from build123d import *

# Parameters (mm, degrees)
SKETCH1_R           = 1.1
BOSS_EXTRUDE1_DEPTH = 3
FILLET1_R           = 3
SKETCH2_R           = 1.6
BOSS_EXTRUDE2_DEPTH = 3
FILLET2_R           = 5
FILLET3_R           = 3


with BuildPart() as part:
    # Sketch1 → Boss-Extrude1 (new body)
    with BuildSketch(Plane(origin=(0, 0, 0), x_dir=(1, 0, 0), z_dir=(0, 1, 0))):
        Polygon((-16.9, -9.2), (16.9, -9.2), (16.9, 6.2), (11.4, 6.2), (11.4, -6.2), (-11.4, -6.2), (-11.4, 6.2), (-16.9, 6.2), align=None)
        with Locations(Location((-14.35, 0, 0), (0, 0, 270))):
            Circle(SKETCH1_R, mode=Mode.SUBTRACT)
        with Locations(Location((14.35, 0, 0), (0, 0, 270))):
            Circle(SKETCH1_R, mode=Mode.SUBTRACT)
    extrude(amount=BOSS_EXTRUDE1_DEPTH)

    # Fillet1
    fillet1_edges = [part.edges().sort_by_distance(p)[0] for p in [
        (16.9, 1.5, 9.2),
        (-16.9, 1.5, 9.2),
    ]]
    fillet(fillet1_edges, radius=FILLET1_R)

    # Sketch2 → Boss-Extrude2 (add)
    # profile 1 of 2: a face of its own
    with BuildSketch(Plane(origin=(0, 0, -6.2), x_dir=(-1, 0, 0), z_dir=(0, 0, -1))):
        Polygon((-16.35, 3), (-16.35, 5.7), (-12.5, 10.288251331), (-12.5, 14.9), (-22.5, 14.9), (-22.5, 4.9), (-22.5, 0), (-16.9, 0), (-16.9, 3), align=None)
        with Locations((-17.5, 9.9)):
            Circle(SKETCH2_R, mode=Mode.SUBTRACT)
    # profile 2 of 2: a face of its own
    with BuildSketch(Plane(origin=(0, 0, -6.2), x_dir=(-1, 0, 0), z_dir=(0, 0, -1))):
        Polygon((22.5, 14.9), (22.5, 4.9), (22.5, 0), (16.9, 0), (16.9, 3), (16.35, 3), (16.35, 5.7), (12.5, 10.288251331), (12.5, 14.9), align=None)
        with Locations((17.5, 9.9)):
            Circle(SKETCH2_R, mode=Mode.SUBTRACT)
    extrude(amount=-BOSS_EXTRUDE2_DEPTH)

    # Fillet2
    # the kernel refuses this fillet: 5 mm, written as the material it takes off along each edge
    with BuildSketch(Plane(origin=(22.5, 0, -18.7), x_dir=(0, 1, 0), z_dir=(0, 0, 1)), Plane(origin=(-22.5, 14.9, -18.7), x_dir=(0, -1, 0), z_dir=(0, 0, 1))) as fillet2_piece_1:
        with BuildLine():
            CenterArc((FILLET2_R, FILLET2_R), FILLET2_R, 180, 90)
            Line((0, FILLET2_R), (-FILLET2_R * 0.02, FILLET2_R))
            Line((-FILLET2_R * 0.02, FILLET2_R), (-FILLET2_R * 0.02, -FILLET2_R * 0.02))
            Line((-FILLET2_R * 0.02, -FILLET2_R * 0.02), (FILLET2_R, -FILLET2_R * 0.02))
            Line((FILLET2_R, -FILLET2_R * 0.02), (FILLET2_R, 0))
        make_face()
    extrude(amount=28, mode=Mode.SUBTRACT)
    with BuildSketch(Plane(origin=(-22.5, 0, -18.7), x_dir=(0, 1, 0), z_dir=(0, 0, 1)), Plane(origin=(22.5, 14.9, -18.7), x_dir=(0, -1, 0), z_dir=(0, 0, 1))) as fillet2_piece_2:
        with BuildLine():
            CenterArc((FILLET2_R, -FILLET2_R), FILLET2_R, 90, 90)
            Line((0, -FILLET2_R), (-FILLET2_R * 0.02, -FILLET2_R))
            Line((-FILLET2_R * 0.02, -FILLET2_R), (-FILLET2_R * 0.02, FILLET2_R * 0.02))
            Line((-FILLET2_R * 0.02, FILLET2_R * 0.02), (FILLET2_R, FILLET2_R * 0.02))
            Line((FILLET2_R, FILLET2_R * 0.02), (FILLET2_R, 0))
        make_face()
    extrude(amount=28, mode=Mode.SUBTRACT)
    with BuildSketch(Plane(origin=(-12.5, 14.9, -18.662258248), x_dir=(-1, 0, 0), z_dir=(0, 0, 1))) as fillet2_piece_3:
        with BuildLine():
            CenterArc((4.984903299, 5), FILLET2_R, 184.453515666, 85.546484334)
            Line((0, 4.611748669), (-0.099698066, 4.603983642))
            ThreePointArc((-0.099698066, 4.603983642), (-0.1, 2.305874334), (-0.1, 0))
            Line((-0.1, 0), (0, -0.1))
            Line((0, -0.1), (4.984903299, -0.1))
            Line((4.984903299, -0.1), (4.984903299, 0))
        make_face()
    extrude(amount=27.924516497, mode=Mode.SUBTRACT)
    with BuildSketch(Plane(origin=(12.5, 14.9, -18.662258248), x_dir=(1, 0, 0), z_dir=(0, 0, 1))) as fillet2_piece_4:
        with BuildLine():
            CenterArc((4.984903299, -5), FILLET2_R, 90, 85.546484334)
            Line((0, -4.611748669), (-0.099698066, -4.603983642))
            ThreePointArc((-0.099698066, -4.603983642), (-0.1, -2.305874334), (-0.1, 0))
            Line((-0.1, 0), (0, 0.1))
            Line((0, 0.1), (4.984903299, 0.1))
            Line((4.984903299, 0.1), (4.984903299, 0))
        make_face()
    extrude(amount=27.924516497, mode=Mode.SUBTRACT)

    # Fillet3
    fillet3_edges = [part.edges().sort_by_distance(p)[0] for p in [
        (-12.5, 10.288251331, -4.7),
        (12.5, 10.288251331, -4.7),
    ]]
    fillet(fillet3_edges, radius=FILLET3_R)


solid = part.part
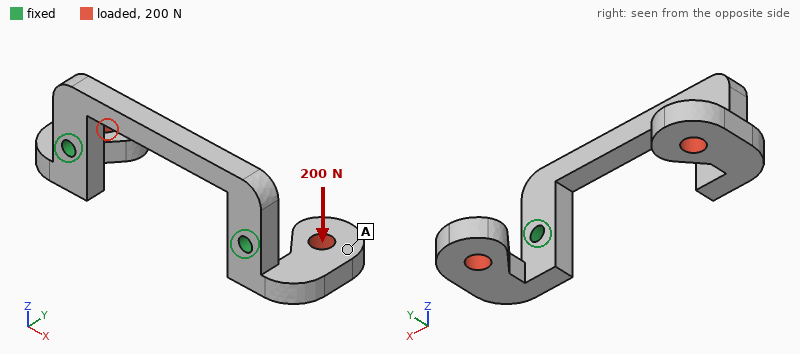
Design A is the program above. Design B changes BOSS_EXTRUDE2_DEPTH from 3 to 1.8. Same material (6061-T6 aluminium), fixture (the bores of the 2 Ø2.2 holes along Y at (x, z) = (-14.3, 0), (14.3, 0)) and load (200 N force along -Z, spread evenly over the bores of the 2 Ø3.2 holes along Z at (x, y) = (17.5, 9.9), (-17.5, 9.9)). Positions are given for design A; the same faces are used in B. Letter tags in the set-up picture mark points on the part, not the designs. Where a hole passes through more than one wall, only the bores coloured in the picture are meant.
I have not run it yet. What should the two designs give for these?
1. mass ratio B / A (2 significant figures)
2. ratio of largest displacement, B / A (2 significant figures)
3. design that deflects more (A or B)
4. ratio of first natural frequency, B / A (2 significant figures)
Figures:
0.82
2.5
B
0.84
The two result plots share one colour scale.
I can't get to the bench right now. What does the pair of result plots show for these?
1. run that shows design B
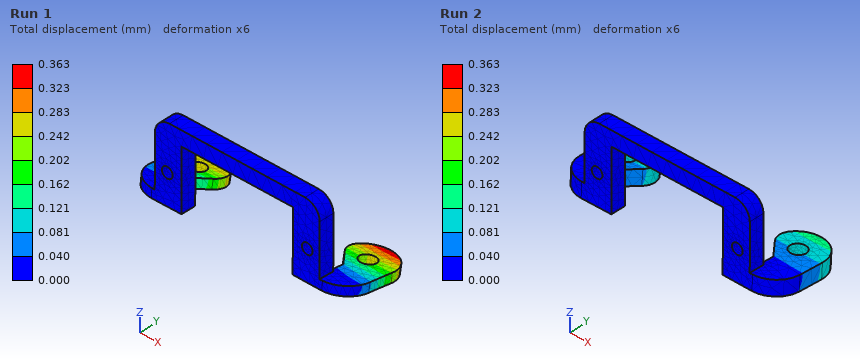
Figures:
Run 1
